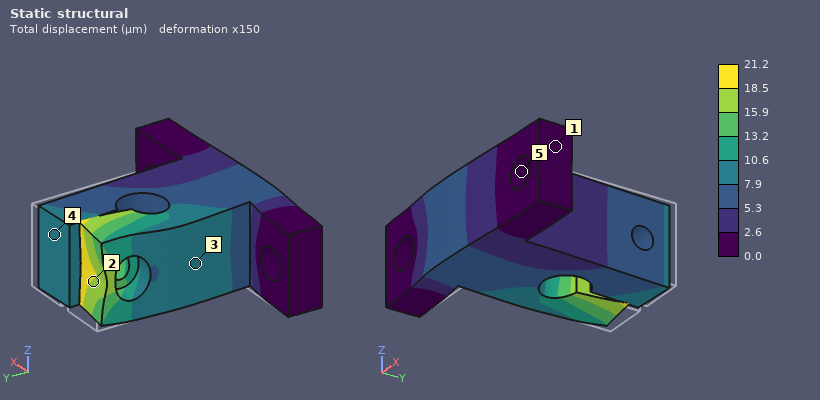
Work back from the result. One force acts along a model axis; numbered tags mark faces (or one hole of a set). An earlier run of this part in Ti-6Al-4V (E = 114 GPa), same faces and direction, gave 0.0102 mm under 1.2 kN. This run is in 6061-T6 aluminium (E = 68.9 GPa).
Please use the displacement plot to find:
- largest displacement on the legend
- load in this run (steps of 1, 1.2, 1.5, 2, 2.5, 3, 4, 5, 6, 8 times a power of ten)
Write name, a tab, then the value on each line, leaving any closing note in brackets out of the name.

largest displacement on the legend	21.2 µm
load in this run	1.5 kN
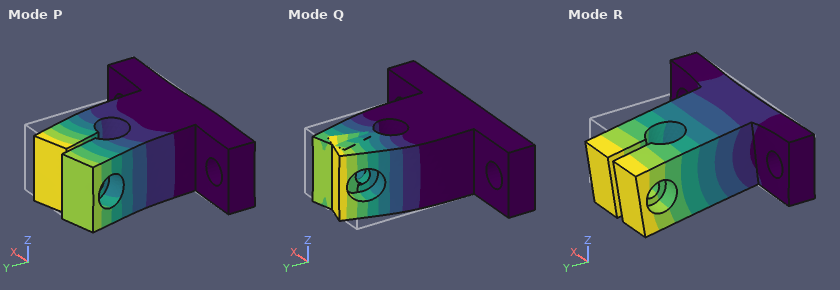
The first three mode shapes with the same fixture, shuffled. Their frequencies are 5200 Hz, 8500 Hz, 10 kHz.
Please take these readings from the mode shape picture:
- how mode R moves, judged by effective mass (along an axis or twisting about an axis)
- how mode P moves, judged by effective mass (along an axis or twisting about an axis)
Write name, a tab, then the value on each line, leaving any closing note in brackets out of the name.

how mode R moves, judged by effective mass	along Z
how mode P moves, judged by effective mass	along X
